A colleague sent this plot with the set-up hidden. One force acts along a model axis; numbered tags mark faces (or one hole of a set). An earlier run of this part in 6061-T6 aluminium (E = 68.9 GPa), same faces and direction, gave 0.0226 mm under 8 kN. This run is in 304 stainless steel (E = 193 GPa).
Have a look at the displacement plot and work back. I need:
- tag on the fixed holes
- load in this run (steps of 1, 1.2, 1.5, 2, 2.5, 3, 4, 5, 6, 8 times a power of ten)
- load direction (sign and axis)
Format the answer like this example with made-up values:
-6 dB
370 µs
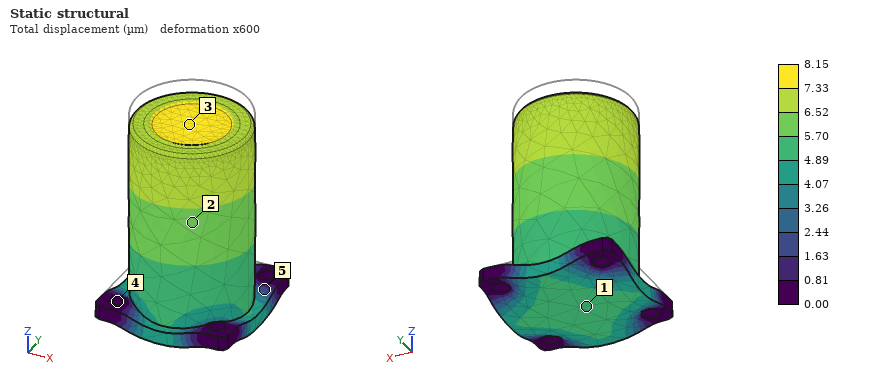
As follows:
4
8 kN
-Z
